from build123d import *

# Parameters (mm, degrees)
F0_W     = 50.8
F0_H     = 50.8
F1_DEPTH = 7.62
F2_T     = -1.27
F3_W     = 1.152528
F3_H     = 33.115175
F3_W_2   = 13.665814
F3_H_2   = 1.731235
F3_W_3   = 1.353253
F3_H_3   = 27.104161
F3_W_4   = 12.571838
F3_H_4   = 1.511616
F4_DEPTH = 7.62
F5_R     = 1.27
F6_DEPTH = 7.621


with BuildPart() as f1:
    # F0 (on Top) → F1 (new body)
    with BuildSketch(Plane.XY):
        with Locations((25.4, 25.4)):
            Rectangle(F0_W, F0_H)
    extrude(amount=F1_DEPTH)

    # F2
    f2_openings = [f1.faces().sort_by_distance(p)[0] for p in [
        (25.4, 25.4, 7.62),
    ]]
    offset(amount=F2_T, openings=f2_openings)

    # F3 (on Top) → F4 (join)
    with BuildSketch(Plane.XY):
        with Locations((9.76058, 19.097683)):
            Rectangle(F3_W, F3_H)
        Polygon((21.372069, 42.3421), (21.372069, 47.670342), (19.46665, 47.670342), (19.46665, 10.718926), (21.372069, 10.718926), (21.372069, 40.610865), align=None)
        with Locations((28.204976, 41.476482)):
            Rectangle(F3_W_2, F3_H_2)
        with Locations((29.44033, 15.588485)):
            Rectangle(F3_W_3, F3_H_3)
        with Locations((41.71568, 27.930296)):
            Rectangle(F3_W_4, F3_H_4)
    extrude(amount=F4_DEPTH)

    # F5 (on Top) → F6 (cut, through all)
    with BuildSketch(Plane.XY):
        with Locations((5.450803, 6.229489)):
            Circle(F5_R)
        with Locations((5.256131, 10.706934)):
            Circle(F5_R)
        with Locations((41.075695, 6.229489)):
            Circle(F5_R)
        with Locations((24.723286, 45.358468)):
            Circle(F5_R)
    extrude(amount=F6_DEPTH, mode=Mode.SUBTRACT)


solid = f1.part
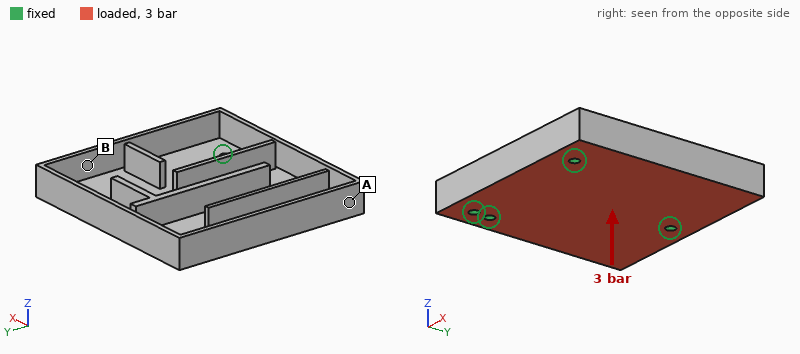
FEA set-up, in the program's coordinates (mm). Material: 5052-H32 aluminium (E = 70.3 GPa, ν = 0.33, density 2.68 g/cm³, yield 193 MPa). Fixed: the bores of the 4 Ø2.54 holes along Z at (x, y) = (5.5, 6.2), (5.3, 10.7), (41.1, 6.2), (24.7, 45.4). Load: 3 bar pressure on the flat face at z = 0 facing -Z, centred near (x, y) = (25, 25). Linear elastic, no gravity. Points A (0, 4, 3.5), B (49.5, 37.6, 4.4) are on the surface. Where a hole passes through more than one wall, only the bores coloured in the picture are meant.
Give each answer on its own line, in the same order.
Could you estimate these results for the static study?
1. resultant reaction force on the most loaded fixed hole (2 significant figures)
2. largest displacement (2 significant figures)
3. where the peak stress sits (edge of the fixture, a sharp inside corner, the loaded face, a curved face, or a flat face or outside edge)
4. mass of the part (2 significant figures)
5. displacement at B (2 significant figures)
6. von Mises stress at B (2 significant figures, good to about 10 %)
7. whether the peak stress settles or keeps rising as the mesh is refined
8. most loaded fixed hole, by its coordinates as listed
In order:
370 N
0.13 mm
edge of the fixture
16 g
0.11 mm
22 MPa
keeps rising
(24.7, 45.4)
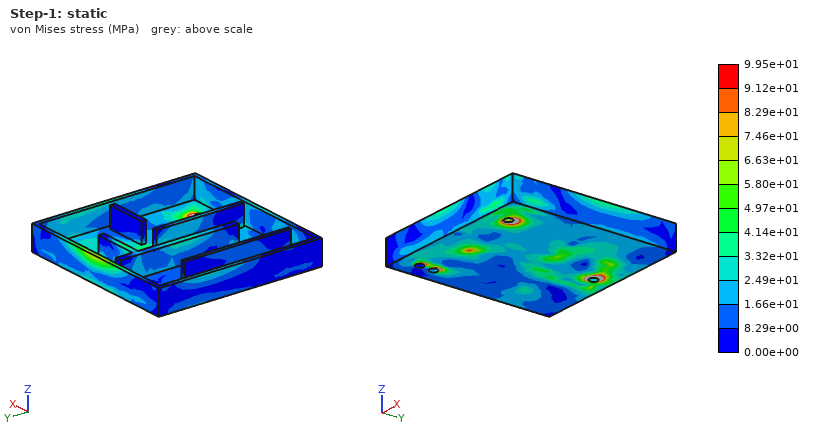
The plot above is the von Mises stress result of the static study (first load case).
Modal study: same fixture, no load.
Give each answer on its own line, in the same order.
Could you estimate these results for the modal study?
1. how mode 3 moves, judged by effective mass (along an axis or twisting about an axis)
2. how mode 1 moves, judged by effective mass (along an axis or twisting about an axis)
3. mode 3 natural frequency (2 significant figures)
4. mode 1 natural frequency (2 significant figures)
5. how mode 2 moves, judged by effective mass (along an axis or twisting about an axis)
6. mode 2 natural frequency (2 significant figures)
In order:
along Z
twisting about Y
5500 Hz
2200 Hz
along Z
5200 Hz
